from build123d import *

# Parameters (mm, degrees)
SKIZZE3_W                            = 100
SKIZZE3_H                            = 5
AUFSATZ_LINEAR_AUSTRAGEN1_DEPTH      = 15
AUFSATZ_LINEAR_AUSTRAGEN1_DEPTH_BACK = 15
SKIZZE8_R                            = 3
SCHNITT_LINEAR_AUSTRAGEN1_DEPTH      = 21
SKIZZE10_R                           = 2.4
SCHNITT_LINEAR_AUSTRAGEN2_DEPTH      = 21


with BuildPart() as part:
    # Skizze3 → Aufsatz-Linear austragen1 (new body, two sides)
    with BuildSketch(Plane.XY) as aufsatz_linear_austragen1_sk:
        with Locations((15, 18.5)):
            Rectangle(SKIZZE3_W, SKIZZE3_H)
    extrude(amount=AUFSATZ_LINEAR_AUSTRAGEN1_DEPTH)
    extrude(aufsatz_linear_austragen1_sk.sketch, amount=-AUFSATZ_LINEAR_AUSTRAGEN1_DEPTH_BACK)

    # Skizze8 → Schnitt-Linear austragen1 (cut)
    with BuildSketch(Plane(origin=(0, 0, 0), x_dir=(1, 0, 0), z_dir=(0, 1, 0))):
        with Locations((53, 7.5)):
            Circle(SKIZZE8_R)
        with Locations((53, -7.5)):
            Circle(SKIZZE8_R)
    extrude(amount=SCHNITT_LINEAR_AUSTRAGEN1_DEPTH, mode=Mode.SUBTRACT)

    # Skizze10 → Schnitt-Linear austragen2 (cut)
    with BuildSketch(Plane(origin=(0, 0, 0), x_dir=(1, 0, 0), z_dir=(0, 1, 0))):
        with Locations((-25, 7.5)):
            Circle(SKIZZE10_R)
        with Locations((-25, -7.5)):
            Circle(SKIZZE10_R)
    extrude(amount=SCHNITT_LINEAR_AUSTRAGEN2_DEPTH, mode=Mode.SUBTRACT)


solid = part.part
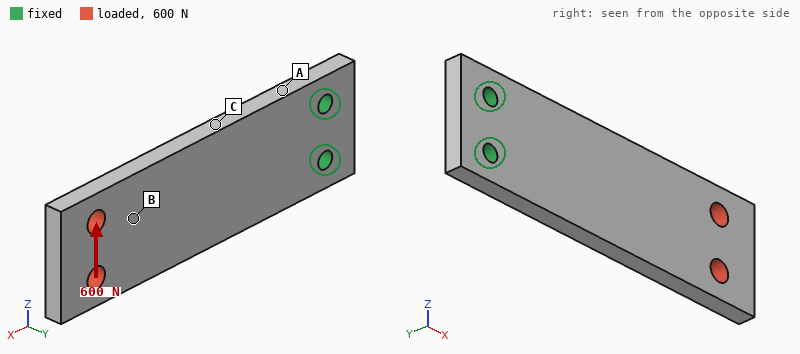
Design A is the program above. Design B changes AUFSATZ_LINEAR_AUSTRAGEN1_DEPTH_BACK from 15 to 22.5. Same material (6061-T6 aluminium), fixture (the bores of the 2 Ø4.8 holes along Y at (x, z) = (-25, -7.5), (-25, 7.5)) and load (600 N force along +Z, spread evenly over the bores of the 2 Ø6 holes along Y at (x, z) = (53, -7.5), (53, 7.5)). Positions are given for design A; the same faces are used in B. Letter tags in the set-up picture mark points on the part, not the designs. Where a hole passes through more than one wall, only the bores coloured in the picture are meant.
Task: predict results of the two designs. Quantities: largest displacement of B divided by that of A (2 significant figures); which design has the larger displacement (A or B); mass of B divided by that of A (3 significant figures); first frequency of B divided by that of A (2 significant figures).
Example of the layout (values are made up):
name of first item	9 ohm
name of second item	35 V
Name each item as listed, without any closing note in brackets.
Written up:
largest displacement of B divided by that of A	0.70
which design has the larger displacement	A
mass of B divided by that of A	1.26
first frequency of B divided by that of A	0.98
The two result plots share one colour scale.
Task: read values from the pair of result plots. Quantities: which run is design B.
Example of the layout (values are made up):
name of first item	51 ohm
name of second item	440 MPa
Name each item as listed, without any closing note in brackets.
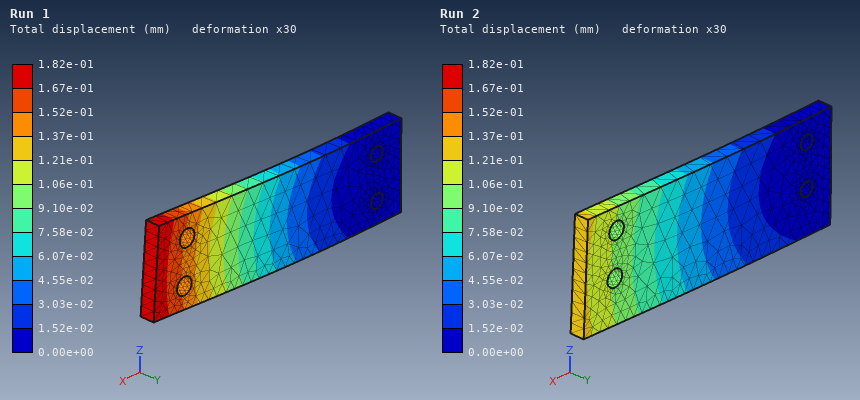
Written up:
which run is design B	Run 2
